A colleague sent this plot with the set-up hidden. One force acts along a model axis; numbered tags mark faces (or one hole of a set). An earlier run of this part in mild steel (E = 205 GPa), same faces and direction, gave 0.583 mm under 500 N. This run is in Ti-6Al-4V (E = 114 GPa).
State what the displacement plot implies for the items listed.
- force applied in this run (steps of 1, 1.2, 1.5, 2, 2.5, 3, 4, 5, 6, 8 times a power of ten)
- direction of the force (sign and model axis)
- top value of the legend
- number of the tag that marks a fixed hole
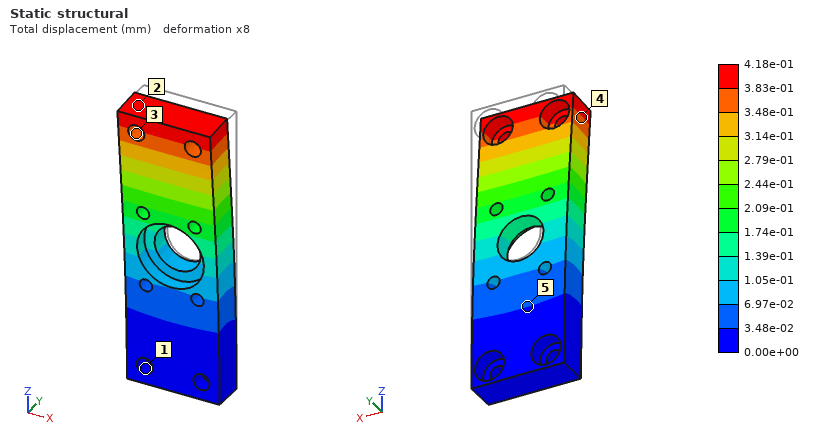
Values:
200 N
-Y
4.18e-01 mm
1
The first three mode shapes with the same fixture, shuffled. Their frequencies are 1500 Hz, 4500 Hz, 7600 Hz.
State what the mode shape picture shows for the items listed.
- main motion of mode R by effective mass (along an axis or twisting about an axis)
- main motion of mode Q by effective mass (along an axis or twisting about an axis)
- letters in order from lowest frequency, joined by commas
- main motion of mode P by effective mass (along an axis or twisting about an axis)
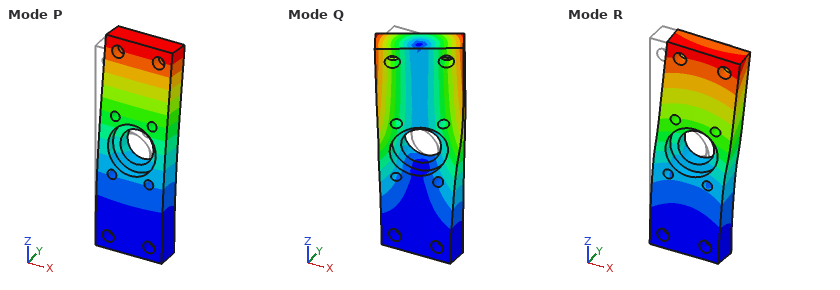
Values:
along X
twisting about Z
P, R, Q
along Y
